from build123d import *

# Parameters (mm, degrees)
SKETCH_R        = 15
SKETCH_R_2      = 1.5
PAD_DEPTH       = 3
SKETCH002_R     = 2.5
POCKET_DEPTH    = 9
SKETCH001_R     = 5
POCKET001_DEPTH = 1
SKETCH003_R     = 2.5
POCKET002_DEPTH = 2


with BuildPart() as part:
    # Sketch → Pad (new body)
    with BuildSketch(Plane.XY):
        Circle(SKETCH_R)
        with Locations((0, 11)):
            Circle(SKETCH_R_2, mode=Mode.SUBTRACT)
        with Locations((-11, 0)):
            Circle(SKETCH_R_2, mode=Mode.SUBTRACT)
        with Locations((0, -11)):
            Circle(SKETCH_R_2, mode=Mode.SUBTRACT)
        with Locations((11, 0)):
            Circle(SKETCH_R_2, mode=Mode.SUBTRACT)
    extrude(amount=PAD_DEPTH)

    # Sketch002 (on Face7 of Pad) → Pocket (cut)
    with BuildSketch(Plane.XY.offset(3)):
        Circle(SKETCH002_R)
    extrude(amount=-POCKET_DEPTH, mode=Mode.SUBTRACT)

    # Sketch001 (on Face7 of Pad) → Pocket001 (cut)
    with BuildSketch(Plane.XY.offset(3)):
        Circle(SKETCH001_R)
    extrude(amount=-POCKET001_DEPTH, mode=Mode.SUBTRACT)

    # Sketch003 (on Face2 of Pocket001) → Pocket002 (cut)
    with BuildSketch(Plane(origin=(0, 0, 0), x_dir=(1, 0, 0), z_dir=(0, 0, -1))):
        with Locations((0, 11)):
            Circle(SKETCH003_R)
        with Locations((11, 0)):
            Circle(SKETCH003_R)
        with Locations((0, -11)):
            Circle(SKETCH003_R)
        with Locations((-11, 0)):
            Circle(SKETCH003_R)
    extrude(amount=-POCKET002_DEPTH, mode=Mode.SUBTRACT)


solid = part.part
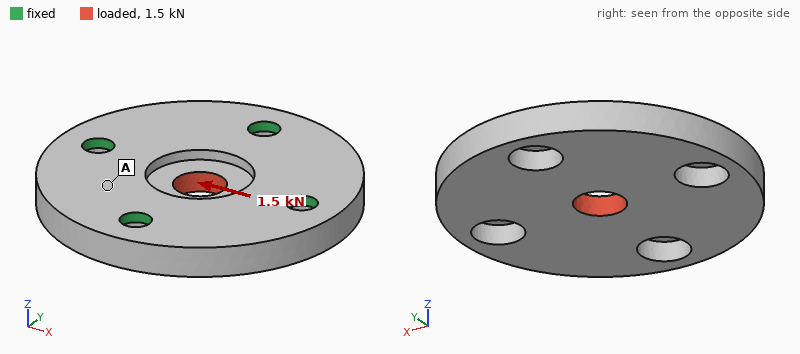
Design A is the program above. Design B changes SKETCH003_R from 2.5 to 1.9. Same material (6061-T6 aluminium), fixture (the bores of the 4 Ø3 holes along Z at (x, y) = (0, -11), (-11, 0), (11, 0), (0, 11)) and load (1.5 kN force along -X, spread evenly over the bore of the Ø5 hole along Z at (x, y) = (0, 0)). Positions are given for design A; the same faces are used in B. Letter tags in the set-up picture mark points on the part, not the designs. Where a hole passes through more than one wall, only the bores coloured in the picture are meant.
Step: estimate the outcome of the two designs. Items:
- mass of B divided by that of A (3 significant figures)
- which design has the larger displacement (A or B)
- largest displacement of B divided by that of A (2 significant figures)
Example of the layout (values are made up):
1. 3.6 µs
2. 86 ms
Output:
1. 1.04
2. A
3. 0.91
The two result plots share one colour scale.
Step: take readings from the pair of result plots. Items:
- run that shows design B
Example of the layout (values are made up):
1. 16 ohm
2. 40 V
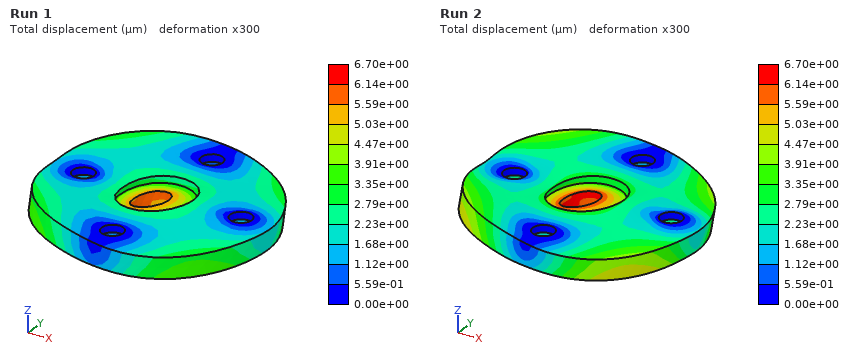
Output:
1. Run 1
